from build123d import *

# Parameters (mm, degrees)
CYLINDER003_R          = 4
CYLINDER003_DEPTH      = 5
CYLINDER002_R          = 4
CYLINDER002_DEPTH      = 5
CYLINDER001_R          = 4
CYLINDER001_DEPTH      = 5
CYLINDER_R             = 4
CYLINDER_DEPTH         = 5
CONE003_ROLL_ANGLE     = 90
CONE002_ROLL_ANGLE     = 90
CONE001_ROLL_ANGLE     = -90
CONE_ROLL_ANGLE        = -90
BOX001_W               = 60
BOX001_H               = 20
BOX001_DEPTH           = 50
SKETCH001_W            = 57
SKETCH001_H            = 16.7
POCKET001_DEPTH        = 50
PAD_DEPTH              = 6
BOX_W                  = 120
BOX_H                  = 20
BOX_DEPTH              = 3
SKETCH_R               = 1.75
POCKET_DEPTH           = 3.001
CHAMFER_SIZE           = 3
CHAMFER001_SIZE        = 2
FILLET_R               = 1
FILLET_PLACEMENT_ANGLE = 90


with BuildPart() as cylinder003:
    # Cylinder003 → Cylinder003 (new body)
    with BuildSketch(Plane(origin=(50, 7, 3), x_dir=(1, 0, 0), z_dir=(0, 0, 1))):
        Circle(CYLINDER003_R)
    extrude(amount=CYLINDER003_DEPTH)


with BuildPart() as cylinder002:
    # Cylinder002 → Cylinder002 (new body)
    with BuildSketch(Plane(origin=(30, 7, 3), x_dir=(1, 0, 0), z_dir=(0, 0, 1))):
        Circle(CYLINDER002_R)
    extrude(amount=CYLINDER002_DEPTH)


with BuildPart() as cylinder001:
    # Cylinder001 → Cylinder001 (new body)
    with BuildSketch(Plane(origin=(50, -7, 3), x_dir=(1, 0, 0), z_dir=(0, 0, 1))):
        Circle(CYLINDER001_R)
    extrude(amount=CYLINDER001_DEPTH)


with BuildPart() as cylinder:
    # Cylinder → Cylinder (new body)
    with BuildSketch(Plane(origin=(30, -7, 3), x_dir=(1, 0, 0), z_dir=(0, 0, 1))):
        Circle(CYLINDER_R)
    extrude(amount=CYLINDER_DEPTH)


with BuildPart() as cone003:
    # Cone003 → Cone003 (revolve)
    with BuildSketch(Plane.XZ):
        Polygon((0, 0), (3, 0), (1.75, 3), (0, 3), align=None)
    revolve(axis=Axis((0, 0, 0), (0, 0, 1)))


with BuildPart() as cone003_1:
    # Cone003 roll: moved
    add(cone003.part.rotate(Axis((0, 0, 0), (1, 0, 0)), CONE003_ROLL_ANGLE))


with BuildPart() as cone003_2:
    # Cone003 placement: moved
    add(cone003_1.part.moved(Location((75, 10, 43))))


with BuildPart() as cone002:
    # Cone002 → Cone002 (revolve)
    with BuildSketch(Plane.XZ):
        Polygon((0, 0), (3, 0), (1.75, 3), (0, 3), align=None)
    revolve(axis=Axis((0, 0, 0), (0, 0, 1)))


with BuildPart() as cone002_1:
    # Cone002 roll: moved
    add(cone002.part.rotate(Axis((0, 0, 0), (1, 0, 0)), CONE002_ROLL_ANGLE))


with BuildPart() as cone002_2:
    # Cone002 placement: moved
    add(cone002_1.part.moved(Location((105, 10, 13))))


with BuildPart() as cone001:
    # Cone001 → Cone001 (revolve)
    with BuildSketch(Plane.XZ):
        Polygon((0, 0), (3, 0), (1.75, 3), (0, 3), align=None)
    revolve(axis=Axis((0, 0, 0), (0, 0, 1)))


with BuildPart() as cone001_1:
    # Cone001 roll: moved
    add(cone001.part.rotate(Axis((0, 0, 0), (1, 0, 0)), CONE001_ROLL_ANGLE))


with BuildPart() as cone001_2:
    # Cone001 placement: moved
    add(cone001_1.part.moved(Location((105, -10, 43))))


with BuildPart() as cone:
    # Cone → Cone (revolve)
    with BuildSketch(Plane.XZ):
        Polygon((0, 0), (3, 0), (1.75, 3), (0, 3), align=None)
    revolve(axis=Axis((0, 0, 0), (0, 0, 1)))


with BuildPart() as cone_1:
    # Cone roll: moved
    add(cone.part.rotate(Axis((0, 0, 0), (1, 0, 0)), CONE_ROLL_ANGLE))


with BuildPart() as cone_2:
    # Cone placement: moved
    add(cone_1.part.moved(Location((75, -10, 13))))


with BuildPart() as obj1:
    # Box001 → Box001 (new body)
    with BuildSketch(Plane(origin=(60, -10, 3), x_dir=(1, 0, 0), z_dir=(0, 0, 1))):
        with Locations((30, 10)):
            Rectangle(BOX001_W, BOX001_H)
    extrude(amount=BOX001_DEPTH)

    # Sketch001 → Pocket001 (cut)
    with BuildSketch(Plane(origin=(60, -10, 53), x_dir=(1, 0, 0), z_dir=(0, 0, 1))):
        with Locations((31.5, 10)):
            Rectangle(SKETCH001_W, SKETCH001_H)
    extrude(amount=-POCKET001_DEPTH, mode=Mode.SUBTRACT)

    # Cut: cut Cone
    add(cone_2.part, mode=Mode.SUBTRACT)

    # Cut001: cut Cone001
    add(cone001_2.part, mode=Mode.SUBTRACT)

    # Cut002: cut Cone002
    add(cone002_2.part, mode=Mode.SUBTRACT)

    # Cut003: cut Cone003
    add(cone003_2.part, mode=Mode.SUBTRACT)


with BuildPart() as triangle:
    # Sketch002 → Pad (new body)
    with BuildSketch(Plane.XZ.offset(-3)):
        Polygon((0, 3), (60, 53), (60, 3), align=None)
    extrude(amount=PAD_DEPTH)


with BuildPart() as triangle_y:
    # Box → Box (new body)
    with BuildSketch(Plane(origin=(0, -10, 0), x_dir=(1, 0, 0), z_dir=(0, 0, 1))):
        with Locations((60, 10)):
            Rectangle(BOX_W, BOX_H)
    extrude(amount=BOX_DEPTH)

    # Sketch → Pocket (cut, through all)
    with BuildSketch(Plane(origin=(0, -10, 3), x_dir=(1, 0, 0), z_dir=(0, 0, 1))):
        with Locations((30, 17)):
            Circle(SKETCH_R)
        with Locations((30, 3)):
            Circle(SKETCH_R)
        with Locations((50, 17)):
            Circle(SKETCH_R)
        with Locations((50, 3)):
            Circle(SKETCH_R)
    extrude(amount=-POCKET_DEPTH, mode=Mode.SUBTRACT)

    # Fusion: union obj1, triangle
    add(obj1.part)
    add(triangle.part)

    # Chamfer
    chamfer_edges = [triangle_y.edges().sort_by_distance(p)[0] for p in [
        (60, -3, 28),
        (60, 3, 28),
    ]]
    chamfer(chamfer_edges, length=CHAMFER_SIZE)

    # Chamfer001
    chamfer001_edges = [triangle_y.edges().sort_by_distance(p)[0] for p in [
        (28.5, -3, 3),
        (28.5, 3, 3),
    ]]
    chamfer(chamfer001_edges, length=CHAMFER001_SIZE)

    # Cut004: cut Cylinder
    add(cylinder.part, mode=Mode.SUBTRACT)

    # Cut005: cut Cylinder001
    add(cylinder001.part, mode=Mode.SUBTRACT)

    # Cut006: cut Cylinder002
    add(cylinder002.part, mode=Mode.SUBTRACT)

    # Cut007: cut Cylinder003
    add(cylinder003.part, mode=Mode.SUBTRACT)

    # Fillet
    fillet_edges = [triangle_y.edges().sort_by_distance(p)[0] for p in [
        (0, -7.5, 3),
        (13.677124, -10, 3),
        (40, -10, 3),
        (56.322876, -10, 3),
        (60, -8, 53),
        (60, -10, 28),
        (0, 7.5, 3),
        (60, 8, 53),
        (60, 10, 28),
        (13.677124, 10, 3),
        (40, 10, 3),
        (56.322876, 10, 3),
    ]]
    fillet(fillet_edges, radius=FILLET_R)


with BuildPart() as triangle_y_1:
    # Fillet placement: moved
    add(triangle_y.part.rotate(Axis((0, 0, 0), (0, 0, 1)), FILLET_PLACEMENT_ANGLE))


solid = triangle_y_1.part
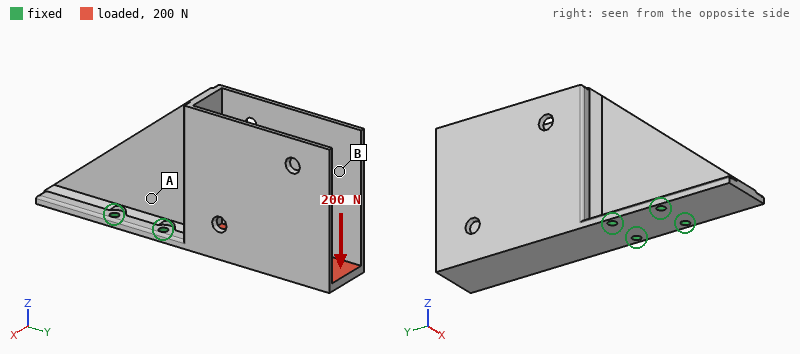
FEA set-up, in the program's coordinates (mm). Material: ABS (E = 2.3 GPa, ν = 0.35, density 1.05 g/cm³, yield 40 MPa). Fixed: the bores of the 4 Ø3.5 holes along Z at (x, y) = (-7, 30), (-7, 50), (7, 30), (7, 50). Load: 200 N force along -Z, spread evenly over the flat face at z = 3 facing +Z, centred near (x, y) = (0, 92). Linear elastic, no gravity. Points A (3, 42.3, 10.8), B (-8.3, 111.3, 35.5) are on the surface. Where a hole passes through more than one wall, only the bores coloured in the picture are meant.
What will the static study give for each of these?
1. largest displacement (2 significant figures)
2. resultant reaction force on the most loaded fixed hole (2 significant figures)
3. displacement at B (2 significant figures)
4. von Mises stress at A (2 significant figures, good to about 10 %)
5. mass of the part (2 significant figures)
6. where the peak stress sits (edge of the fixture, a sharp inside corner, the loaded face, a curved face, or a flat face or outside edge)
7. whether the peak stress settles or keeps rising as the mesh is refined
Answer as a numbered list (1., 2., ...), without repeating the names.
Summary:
1. 1.1 mm
2. 300 N
3. 0.89 mm
4. 4.3 MPa
5. 30 g
6. edge of the fixture
7. keeps rising
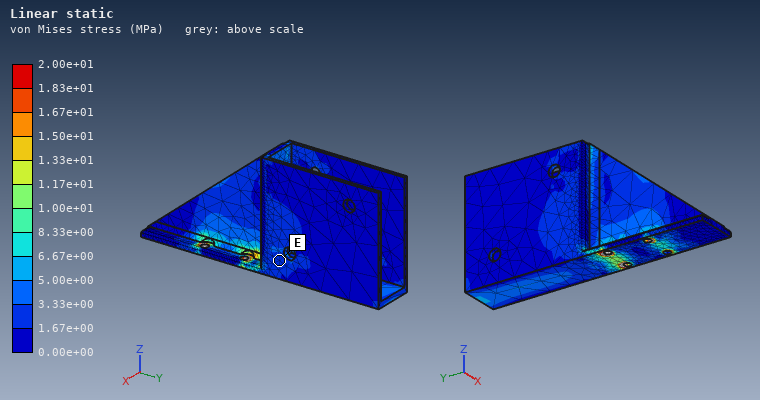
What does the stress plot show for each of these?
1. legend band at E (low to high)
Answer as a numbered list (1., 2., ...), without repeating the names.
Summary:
1. 1.67e+00 to 3.33e+00 MPa
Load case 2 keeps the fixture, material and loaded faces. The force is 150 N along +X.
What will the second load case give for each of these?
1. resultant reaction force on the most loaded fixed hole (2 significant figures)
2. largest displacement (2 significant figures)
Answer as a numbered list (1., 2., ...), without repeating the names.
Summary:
1. 380 N
2. 1.5 mm
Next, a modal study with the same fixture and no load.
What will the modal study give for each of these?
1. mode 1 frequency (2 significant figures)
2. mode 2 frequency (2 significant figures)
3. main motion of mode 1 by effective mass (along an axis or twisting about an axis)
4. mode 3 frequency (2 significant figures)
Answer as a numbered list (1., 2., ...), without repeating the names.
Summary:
1. 250 Hz
2. 270 Hz
3. along X
4. 610 Hz
